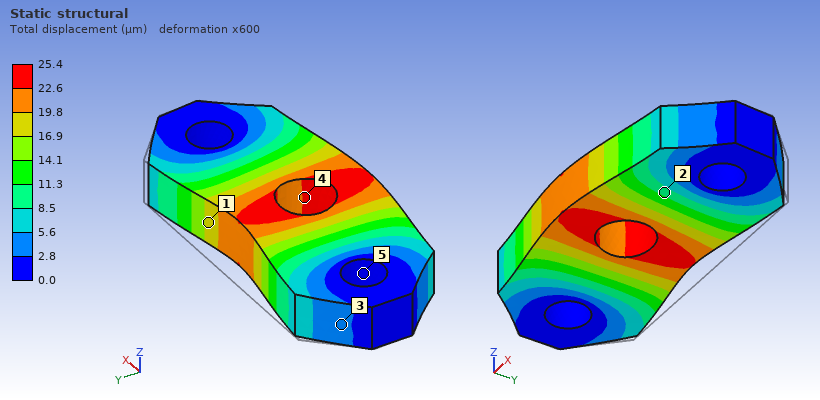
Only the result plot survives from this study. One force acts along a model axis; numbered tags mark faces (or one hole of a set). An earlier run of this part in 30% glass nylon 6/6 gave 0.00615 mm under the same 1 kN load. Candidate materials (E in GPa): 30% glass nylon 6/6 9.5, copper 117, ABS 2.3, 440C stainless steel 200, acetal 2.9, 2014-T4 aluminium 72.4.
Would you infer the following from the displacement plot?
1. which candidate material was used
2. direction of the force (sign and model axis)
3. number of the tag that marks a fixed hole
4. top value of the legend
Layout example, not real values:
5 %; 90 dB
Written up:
ABS; -Y; 5; 25.4 µm
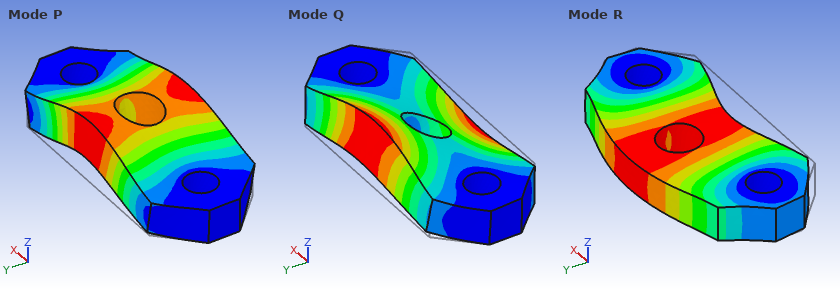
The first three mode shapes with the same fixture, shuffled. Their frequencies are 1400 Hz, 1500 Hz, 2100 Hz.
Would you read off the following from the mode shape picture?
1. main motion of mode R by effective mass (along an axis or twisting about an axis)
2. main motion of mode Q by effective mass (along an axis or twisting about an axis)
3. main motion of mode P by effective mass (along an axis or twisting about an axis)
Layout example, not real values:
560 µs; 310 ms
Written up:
along Y; twisting about X; along Z
